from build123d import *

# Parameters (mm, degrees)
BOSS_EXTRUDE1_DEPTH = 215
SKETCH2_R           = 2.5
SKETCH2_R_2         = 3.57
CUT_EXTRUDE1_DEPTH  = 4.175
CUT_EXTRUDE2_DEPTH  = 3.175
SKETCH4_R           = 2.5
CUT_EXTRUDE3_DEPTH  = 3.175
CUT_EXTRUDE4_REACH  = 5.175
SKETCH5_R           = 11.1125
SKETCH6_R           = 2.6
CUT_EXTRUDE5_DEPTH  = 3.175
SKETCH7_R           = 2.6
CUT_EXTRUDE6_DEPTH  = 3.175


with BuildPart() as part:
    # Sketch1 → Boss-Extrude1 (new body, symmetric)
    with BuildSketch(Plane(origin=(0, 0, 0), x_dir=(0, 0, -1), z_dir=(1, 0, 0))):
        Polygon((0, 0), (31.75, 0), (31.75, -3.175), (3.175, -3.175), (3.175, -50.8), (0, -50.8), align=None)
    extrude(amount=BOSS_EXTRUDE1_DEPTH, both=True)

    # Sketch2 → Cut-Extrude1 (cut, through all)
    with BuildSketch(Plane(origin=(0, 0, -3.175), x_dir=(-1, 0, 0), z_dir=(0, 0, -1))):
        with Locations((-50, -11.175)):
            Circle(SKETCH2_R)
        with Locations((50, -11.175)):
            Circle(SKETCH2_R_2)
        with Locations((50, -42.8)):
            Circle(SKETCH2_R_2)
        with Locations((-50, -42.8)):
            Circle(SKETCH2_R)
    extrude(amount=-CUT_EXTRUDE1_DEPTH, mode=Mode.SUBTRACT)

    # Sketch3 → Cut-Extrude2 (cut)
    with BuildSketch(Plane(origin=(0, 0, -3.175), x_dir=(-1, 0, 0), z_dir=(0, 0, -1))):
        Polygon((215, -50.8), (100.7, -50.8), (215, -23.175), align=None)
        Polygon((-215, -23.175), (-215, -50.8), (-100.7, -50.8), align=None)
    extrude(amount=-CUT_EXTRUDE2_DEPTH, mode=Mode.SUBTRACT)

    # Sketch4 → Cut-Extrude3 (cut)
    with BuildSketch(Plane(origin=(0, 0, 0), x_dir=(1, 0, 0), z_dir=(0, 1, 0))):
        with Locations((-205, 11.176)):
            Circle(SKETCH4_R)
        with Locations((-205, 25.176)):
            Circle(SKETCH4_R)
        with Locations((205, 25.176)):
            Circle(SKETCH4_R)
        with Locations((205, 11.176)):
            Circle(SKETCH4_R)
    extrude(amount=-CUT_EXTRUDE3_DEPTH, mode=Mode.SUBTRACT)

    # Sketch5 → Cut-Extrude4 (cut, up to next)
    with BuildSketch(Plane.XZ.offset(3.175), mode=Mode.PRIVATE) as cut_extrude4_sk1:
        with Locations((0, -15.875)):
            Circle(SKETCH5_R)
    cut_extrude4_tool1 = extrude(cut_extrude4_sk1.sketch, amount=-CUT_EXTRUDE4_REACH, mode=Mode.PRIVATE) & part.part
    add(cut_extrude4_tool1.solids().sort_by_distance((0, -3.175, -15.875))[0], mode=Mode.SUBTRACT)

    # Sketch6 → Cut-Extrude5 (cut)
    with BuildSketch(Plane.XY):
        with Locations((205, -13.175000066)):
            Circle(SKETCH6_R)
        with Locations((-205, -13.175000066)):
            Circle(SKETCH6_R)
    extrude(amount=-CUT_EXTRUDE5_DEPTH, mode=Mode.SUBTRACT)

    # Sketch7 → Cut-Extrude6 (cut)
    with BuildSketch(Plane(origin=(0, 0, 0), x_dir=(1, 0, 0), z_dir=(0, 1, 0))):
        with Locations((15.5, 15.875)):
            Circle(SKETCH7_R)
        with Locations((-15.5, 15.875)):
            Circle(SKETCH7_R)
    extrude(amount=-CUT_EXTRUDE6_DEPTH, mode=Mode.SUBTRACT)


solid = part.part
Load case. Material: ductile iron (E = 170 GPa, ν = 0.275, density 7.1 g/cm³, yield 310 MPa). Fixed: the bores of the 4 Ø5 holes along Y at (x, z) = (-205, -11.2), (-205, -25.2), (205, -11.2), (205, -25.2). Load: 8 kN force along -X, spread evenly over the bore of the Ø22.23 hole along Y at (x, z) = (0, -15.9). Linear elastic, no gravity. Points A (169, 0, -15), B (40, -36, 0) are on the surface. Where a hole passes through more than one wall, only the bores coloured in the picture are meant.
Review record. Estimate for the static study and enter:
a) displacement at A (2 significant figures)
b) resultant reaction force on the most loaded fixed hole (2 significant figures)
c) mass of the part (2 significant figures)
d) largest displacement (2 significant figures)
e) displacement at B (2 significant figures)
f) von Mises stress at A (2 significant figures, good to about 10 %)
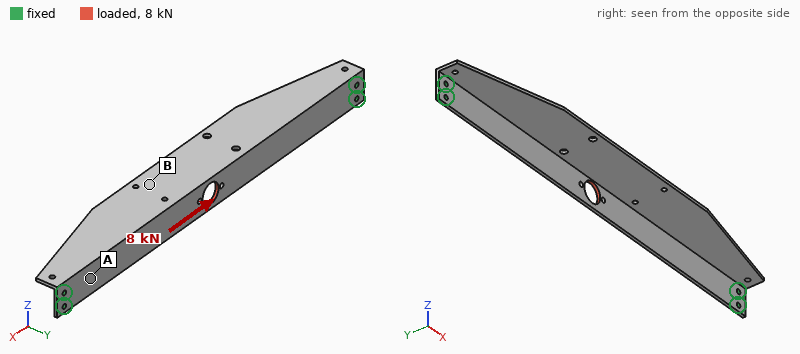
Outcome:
17 µm
3.2 kN
680 g
45 µm
26 µm
35 MPa
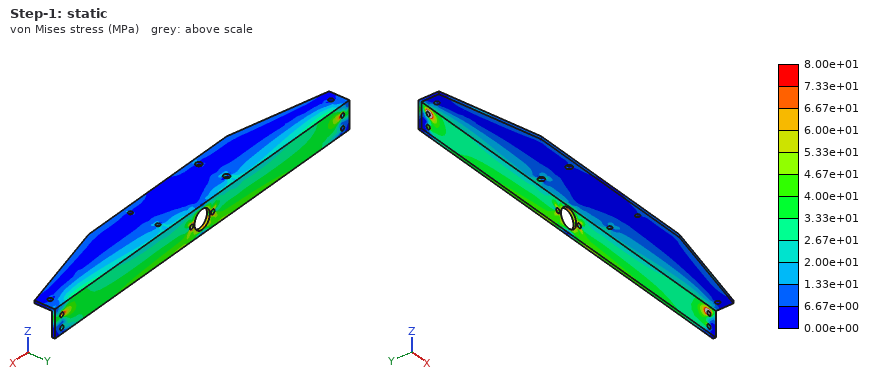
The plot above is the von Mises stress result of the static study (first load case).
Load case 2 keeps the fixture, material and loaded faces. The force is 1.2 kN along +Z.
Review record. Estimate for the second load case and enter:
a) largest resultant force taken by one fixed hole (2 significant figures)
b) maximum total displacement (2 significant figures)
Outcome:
3.4 kN
0.27 mm
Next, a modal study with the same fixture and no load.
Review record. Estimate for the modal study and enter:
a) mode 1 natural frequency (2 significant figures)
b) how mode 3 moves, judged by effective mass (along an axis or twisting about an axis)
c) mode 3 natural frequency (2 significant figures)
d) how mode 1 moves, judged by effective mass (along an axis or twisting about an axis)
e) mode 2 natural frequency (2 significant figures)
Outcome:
260 Hz
along Y
630 Hz
along Z
570 Hz
